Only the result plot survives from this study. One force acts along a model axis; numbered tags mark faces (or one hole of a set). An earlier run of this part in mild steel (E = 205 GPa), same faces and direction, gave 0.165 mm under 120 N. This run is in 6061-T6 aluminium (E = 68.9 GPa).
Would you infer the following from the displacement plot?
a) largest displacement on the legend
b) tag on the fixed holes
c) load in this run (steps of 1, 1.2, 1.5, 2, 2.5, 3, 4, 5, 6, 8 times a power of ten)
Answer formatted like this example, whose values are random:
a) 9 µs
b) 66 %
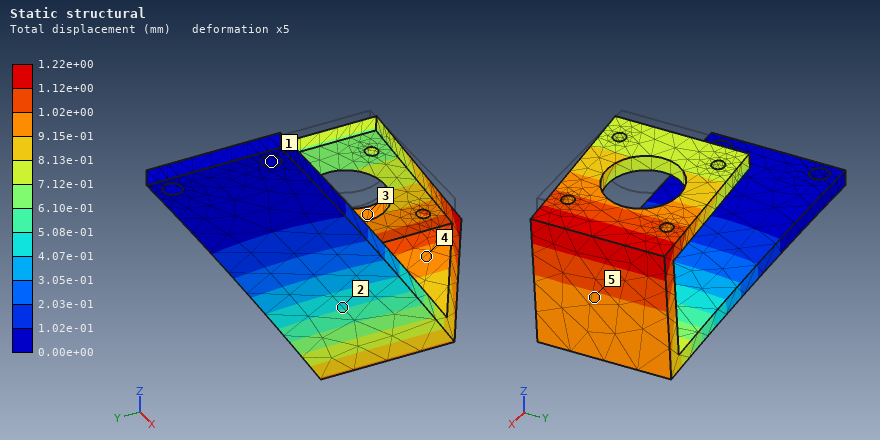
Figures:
a) 1.22e+00 mm
b) 1
c) 300 N
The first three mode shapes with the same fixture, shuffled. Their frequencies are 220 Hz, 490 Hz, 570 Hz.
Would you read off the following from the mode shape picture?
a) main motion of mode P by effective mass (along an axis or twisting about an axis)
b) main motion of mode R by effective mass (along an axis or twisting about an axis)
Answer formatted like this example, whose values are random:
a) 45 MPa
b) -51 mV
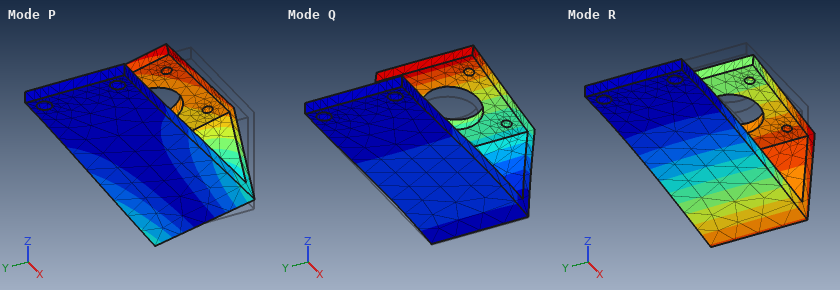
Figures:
a) along Y
b) along Z
